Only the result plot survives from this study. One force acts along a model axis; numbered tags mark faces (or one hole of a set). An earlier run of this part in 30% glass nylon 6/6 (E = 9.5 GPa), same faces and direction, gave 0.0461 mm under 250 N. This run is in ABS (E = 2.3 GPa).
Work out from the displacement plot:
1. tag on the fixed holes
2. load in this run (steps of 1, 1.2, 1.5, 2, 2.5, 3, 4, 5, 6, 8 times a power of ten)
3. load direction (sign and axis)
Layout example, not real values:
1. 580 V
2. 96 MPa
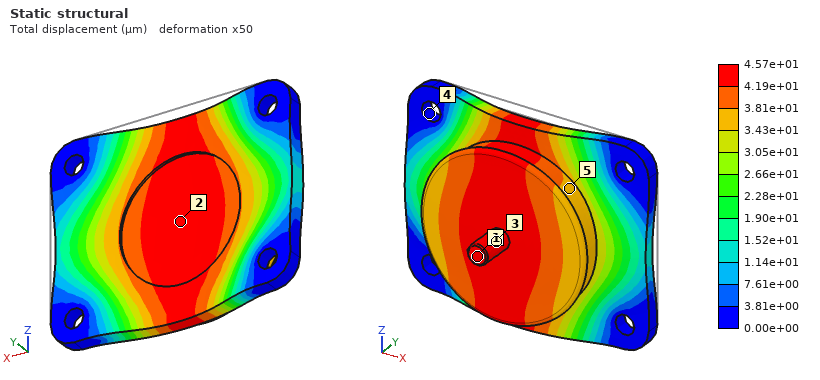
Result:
1. 4
2. 60 N
3. -Y
